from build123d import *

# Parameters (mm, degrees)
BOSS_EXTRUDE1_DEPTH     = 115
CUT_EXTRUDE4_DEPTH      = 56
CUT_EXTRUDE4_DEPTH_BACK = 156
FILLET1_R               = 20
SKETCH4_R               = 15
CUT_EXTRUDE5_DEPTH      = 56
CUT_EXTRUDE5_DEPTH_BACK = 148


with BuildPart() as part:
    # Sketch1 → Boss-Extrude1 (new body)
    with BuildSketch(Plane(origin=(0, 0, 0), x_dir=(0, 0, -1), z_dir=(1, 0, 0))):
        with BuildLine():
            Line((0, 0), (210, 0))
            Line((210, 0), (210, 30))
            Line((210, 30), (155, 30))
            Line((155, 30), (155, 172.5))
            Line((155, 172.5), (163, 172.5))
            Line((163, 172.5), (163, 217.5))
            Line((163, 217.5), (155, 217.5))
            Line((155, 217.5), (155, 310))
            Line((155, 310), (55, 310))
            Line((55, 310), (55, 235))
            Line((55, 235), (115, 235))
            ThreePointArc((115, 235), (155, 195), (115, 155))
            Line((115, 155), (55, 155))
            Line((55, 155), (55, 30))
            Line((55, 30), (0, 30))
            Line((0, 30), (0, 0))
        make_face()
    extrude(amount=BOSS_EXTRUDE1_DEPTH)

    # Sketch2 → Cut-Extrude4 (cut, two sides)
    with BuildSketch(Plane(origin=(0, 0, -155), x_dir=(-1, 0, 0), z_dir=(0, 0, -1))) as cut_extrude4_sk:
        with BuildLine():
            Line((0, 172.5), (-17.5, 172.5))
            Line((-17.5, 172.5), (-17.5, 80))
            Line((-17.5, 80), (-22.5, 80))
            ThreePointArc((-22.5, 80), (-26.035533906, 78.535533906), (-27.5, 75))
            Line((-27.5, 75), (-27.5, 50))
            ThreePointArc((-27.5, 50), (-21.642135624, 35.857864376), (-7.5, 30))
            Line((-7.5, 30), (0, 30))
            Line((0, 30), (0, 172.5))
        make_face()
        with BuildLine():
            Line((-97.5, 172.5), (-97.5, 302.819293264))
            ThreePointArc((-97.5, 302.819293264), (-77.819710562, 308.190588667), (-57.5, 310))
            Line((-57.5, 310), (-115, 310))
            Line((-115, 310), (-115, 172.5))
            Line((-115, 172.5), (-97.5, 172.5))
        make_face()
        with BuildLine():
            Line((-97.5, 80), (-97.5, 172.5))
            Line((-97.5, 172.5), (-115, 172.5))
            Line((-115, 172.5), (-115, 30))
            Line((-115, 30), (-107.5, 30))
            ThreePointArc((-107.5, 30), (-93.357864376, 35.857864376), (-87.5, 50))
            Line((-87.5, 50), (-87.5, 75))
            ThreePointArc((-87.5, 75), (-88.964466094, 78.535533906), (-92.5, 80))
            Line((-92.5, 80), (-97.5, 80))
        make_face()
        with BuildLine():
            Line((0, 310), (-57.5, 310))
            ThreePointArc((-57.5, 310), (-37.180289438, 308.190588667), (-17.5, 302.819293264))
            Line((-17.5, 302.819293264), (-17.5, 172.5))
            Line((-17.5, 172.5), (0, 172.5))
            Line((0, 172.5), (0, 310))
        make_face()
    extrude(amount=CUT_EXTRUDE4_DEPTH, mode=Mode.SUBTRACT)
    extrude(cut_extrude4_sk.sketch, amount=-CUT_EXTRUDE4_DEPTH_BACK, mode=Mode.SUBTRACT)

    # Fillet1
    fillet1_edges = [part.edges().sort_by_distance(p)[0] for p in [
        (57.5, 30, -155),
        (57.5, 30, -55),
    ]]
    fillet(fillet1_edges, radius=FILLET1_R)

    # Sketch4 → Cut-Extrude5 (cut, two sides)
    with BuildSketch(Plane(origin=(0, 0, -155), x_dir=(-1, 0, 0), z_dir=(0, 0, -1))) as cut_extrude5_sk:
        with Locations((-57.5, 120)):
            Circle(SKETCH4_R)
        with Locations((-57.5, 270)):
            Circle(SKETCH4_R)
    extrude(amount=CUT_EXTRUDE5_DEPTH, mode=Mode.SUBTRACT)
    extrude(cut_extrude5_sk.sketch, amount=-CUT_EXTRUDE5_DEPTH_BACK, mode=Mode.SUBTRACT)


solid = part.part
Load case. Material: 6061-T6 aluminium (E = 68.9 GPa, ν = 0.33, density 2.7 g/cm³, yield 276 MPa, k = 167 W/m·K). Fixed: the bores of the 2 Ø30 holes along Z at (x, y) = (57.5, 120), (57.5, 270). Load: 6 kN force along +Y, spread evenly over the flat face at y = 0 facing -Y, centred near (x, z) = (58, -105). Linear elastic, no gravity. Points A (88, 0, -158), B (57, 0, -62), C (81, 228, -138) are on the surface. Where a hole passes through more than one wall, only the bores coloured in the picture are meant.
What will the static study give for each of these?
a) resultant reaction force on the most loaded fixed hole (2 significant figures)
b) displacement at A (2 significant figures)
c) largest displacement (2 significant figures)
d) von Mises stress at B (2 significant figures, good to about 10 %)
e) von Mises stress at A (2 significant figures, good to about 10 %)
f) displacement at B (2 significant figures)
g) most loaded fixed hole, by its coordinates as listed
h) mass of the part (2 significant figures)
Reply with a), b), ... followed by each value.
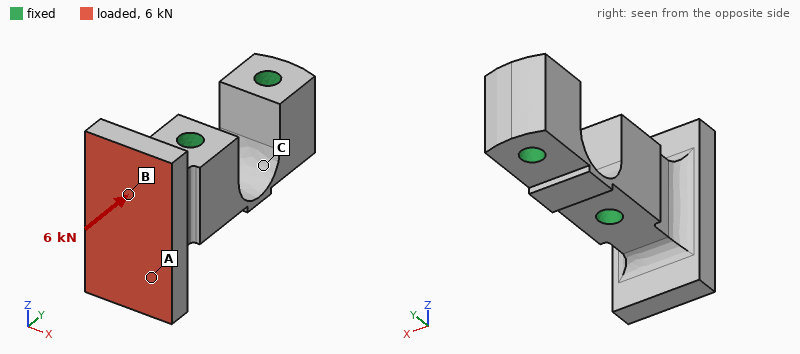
a) 6.0 kN
b) 2.4 µm
c) 6.1 µm
d) 1.7 MPa
e) 1.5 MPa
f) 1.8 µm
g) (57.5, 120)
h) 5.9 kg
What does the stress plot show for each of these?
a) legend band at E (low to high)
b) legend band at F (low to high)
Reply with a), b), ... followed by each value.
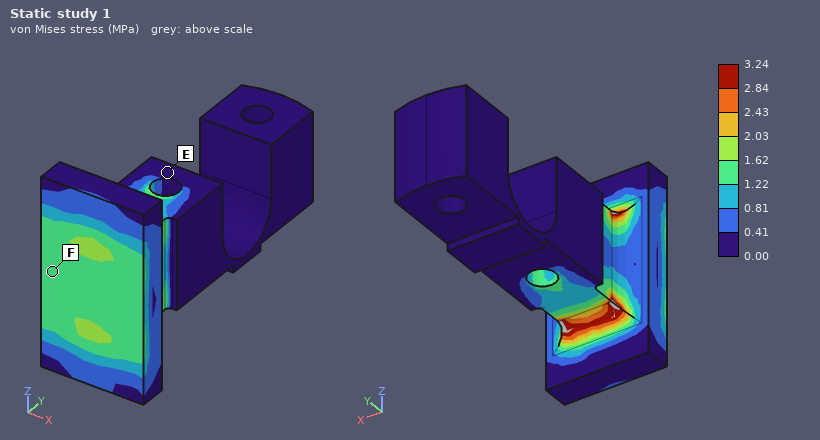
a) 0.00 to 0.41 MPa
b) 1.22 to 1.62 MPa
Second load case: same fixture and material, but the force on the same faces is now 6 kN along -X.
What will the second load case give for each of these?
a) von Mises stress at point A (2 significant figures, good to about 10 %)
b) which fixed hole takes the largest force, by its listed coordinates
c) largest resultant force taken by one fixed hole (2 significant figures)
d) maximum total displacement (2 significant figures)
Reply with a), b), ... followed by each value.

a) 1.3 MPa
b) (57.5, 120)
c) 6.4 kN
d) 34 µm
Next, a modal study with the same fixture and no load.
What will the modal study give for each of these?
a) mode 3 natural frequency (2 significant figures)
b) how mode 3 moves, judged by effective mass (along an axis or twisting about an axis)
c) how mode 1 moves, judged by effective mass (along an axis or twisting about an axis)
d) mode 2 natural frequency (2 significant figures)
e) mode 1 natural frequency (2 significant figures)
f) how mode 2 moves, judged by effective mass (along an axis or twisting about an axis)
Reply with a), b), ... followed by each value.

a) 2300 Hz
b) along Z
c) along X
d) 2100 Hz
e) 1700 Hz
f) twisting about Y
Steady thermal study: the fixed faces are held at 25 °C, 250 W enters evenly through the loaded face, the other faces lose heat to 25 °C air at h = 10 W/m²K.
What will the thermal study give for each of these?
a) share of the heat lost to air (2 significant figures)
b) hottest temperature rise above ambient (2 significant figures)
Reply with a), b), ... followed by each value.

a) 4.2 %
b) 24 K
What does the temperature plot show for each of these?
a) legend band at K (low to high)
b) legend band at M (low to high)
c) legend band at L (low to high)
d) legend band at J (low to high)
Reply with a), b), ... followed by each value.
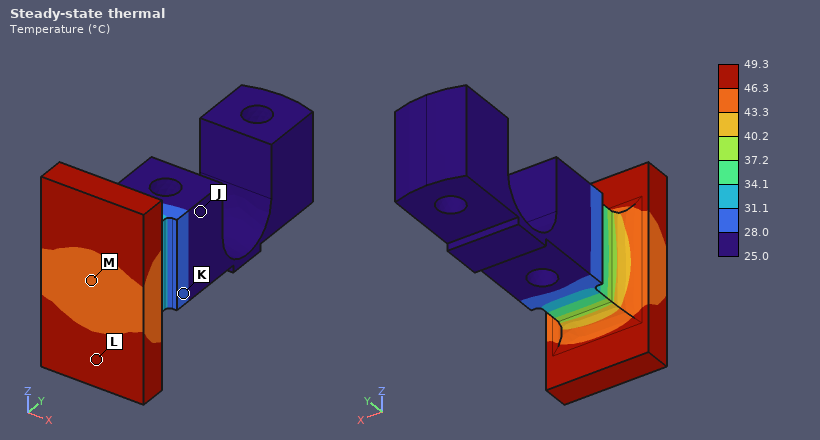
a) 28.0 to 31.1 °C
b) 43.3 to 46.3 °C
c) 46.3 to 49.3 °C
d) 25.0 to 28.0 °C
